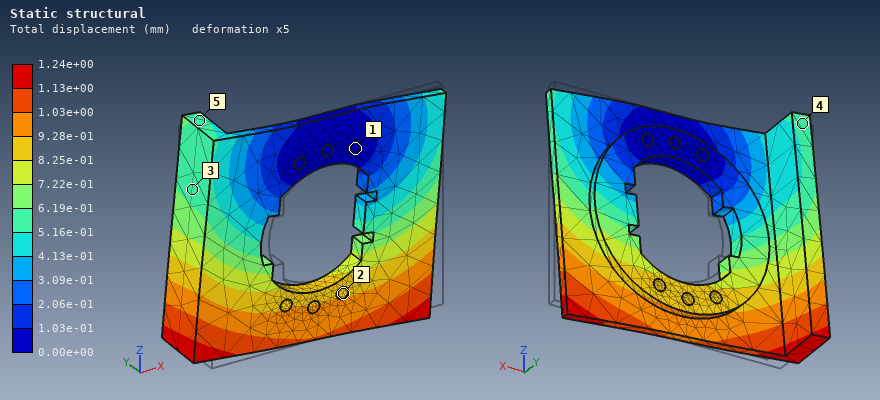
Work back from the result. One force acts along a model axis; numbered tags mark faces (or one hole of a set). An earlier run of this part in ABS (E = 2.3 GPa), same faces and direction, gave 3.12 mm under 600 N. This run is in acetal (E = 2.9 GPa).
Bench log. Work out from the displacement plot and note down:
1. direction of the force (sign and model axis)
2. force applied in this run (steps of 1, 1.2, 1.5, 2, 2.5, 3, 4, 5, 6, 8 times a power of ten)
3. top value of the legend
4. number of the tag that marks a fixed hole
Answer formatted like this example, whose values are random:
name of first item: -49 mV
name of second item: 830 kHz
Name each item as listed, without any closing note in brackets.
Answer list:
direction of the force: -X
force applied in this run: 300 N
top value of the legend: 1.24e+00 mm
number of the tag that marks a fixed hole: 1
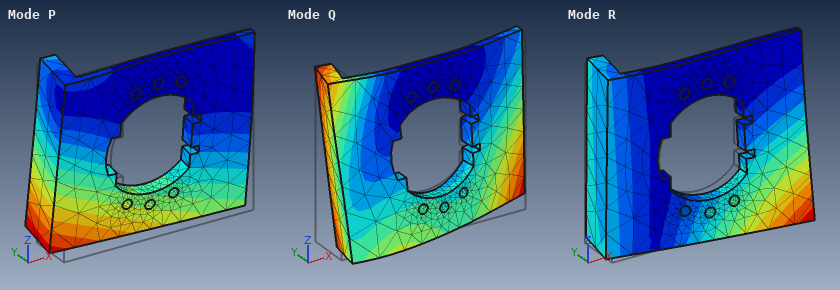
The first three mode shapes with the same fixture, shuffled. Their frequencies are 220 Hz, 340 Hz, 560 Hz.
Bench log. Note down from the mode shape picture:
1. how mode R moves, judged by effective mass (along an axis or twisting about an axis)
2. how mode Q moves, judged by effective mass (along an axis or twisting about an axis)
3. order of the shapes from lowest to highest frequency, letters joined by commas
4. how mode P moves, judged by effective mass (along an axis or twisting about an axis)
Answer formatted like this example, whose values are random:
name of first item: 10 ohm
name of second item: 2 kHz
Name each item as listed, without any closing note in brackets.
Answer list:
how mode R moves, judged by effective mass: twisting about Z
how mode Q moves, judged by effective mass: along X
order of the shapes from lowest to highest frequency, letters joined by commas: P, R, Q
how mode P moves, judged by effective mass: along Y
